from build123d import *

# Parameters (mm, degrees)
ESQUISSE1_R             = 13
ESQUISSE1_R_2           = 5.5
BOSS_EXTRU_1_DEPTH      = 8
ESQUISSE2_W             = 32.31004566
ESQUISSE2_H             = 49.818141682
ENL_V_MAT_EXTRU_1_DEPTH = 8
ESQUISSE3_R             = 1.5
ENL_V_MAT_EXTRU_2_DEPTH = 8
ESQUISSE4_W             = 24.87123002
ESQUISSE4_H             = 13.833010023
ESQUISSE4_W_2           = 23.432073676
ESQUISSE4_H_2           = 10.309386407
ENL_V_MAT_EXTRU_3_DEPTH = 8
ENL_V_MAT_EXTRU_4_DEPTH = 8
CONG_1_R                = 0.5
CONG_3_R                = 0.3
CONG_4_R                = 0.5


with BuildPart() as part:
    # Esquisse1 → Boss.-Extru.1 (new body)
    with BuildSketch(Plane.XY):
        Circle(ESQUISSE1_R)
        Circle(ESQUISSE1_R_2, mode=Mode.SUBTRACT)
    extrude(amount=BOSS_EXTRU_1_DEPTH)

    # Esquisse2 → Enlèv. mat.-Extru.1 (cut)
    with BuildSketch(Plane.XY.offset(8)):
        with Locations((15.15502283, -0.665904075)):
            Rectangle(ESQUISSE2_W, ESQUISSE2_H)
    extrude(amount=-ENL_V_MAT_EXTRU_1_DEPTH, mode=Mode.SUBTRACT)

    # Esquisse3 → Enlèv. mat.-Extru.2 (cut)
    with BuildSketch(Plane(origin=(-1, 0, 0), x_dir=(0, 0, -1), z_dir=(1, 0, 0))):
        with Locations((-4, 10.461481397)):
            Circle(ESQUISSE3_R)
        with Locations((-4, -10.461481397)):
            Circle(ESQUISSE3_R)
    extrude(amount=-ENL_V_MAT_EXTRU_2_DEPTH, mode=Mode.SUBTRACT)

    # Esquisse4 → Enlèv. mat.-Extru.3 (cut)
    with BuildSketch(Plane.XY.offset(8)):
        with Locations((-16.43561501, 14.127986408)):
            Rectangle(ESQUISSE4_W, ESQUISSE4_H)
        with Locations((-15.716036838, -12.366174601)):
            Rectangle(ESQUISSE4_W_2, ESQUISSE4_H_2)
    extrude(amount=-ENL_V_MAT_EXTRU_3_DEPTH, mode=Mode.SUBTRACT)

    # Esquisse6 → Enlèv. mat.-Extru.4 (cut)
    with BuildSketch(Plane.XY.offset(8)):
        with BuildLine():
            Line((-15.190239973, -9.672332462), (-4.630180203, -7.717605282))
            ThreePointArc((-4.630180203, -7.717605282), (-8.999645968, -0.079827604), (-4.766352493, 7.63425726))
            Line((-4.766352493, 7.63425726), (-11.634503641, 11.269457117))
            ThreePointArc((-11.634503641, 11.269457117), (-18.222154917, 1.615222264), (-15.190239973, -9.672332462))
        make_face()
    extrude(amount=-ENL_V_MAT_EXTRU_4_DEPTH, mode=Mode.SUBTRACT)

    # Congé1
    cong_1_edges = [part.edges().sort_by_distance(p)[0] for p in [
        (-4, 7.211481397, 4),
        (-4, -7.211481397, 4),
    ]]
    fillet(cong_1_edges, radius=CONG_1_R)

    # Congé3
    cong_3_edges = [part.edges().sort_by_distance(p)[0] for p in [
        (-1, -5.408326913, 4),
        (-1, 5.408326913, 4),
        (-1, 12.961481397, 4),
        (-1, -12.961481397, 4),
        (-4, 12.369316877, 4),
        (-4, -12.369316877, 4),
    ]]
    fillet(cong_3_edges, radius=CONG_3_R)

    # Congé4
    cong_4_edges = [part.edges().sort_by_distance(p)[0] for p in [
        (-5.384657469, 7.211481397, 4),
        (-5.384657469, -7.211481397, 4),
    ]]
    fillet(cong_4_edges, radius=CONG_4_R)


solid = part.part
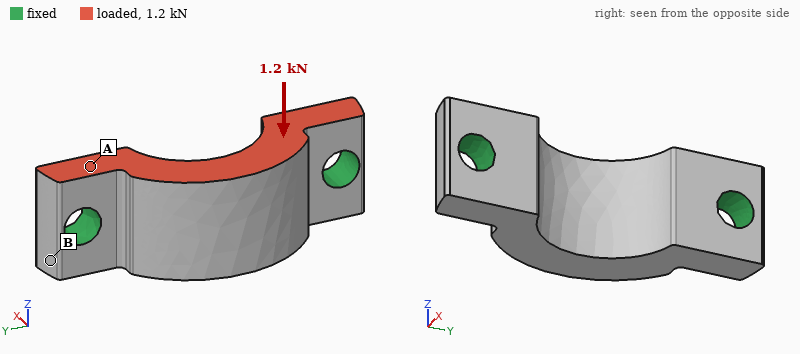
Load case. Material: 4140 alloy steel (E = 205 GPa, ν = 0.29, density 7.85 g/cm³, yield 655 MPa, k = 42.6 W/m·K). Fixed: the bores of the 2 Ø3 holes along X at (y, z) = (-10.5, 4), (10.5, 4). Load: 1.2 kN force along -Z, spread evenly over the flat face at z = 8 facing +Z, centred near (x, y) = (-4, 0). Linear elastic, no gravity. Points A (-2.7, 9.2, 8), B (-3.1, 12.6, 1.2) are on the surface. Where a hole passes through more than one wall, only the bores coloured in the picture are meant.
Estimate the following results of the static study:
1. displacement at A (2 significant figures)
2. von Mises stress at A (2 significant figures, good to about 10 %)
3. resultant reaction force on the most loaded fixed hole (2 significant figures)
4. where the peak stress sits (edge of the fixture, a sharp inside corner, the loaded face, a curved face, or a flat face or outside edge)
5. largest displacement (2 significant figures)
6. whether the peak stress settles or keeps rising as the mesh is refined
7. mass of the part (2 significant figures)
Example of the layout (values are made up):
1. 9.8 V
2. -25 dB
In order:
1. 1.7 µm
2. 68 MPa
3. 600 N
4. edge of the fixture
5. 9.4 µm
6. keeps rising
7. 5.7 g
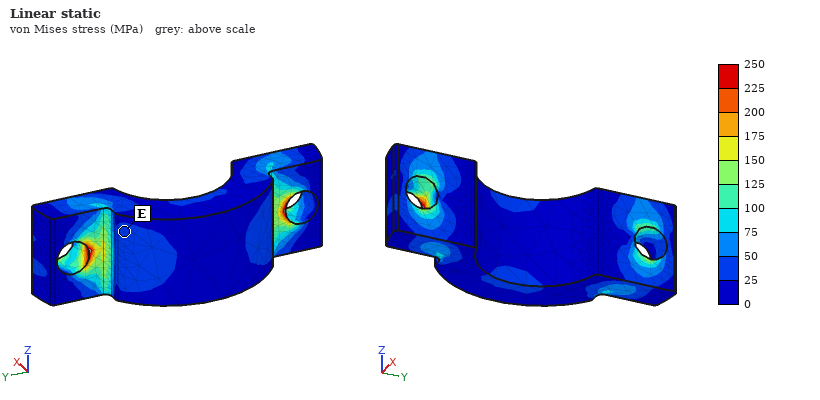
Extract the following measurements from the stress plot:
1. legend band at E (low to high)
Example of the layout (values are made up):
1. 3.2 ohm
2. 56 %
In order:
1. 25 to 50 MPa
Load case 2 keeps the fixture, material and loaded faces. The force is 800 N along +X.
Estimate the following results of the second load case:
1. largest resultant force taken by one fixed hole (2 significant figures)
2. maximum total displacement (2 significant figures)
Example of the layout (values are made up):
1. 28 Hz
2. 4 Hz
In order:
1. 450 N
2. 8.1 µm
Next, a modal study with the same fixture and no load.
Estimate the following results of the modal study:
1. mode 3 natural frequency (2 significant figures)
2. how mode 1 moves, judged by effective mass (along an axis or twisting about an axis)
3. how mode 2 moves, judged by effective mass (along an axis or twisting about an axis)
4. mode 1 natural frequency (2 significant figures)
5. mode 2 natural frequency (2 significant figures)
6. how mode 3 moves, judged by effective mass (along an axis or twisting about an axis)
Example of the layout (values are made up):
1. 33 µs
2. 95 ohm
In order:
1. 67 kHz
2. along Z
3. along X
4. 28 kHz
5. 51 kHz
6. along Y
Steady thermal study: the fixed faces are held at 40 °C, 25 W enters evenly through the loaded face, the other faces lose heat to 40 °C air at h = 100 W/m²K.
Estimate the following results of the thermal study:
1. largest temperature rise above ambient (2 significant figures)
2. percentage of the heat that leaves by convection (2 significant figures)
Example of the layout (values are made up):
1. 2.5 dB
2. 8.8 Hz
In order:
1. 68 K
2. 6.9 %
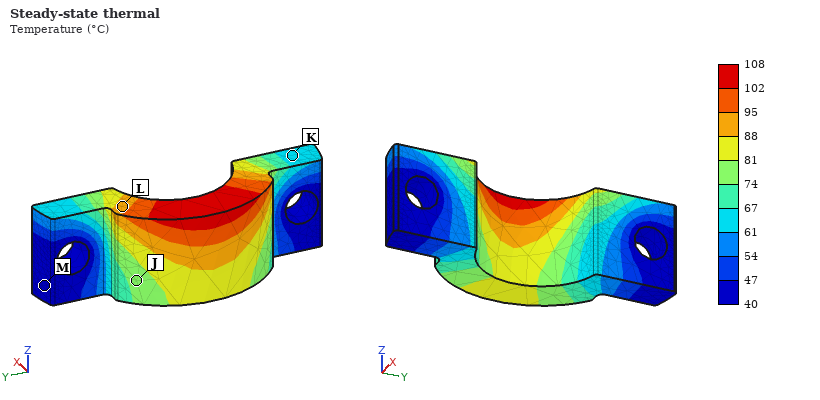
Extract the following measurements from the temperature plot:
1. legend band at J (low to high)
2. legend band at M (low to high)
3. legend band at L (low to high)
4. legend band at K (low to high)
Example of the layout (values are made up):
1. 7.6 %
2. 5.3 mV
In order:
1. 74 to 81 °C
2. 40 to 47 °C
3. 88 to 95 °C
4. 61 to 67 °C
